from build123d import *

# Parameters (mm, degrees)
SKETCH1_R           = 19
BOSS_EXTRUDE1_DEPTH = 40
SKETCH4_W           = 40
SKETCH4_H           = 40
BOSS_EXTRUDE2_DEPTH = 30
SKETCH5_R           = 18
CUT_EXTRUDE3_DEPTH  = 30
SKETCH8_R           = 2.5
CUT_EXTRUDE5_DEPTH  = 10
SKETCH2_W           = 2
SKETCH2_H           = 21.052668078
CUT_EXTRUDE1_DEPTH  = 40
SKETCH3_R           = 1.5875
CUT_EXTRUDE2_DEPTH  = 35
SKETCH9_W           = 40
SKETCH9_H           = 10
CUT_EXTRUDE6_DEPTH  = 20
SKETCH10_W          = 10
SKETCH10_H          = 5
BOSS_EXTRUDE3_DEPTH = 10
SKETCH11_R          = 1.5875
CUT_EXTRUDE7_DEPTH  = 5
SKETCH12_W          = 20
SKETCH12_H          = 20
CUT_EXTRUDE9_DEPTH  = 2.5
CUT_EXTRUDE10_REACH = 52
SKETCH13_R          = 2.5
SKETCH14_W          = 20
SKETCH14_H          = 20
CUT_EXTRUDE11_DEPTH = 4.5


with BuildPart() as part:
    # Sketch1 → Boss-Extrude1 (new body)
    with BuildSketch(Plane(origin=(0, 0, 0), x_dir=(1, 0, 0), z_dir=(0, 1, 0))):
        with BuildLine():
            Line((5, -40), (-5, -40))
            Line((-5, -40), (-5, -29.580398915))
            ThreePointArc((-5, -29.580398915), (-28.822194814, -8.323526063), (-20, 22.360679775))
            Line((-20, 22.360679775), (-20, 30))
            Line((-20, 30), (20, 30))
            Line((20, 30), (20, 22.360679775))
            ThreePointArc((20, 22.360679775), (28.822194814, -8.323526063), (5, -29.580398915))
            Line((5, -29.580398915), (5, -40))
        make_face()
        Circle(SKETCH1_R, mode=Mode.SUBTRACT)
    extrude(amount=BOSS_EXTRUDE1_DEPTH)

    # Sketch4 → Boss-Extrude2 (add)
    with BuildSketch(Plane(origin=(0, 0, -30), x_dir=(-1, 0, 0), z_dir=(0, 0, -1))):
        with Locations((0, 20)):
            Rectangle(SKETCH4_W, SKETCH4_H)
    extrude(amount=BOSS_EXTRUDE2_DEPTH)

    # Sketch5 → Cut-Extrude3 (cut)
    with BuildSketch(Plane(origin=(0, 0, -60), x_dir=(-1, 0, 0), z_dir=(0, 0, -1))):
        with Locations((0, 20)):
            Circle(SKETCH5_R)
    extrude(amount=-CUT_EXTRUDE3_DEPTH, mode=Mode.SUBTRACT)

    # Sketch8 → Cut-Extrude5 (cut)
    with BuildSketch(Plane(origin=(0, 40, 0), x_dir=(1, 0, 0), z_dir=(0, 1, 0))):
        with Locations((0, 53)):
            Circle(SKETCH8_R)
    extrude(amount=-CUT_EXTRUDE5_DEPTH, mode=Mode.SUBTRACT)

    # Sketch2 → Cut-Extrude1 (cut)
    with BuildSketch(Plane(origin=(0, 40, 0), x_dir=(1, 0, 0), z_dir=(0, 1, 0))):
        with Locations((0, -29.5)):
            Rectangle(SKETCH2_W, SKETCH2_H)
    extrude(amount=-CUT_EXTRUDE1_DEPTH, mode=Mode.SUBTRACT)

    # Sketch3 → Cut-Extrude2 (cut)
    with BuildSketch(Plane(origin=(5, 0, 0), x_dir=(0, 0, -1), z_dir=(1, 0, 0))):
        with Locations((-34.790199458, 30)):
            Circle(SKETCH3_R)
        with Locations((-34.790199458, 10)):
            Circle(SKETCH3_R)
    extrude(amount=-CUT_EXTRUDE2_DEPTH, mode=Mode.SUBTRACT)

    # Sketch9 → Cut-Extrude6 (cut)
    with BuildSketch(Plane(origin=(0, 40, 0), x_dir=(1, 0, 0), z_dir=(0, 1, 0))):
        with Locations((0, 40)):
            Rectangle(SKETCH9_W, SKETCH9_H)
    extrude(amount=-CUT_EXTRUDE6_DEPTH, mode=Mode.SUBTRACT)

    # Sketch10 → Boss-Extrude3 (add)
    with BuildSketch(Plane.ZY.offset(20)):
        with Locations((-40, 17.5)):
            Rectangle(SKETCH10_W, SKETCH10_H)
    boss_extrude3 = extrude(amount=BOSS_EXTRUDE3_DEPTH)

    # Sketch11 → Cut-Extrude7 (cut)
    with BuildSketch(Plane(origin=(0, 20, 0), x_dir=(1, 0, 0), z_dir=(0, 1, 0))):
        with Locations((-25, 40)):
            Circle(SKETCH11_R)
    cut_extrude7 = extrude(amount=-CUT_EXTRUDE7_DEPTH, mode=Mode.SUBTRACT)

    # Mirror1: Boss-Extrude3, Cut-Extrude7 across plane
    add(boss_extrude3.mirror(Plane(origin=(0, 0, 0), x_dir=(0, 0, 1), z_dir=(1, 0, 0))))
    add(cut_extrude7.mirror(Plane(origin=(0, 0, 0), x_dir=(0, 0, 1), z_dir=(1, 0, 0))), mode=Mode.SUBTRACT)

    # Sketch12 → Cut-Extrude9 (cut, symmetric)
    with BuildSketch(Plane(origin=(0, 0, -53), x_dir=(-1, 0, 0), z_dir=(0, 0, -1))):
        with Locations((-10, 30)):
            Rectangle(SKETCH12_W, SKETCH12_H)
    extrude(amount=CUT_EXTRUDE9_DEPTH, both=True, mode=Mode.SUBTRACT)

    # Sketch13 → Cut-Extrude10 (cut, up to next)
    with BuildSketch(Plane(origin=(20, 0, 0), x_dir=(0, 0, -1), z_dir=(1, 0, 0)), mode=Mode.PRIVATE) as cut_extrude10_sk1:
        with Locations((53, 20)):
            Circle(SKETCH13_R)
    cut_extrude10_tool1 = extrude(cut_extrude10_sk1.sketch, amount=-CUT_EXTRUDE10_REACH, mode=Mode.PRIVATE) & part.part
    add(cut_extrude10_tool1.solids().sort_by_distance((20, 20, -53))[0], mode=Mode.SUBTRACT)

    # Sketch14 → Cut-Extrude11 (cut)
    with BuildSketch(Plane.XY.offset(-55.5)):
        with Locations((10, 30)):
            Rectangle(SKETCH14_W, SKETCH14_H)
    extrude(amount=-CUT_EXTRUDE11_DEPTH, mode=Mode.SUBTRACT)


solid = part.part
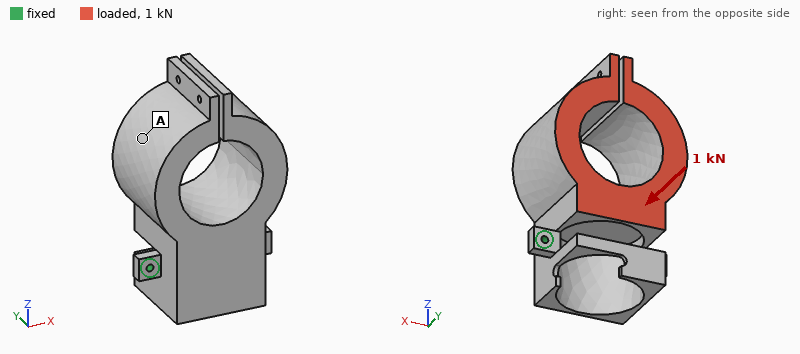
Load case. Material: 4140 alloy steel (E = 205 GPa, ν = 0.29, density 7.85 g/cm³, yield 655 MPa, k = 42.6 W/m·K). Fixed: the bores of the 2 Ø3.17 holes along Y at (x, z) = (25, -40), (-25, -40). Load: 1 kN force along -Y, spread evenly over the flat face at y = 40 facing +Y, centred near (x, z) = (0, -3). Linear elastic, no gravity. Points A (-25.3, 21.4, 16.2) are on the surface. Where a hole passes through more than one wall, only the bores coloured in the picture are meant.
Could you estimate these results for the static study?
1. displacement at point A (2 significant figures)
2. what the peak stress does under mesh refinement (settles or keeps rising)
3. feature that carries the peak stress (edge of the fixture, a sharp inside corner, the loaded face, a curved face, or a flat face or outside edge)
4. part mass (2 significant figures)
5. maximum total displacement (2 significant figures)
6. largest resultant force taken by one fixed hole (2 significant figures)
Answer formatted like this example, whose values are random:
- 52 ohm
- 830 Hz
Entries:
- 0.27 mm
- keeps rising
- edge of the fixture
- 690 g
- 0.40 mm
- 520 N
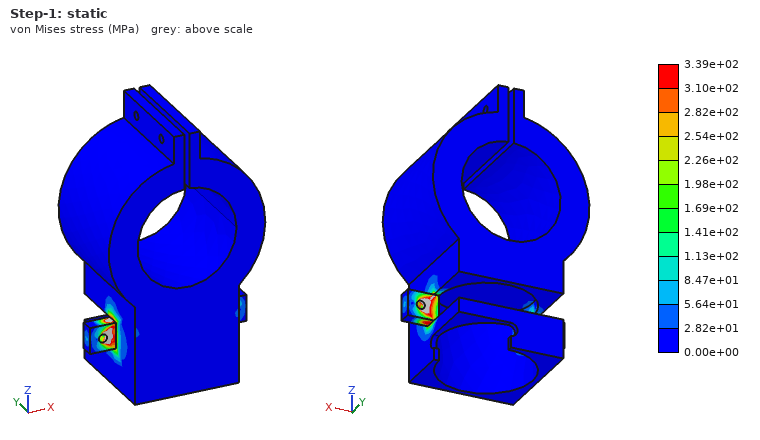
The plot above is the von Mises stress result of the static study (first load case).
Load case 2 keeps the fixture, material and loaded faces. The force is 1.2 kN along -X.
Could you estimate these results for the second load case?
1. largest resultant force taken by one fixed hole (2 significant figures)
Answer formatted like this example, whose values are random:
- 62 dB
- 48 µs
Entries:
- 1.3 kN
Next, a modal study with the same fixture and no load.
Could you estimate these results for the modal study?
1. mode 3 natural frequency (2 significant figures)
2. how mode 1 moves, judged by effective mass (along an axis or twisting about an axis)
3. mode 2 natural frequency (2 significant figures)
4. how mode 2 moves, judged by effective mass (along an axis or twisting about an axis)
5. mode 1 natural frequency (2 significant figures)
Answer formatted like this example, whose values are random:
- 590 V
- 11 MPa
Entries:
- 2000 Hz
- along Y
- 1500 Hz
- along X
- 390 Hz
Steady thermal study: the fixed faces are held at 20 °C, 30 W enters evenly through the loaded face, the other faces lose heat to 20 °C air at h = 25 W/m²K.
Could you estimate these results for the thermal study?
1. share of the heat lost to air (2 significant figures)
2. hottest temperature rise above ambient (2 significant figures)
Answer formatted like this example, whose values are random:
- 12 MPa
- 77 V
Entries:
- 67 %
- 47 K
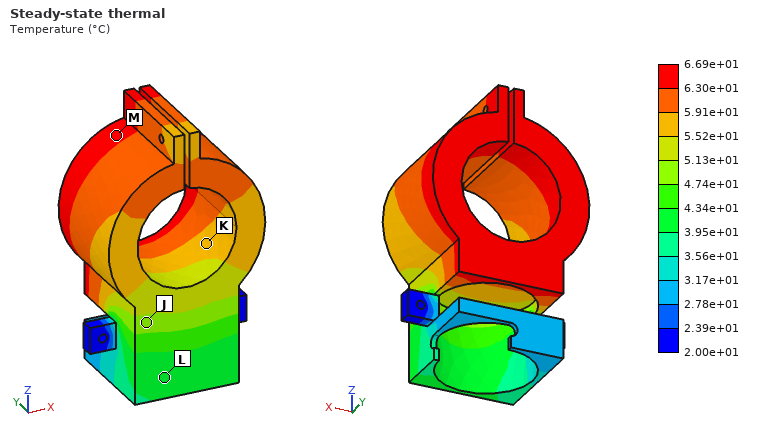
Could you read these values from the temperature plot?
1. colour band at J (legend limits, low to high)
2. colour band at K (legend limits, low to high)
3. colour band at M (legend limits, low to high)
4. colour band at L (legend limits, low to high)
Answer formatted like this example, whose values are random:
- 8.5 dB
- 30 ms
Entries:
- 4.74e+01 to 5.13e+01 °C
- 5.52e+01 to 5.91e+01 °C
- 6.30e+01 to 6.69e+01 °C
- 3.95e+01 to 4.34e+01 °C
